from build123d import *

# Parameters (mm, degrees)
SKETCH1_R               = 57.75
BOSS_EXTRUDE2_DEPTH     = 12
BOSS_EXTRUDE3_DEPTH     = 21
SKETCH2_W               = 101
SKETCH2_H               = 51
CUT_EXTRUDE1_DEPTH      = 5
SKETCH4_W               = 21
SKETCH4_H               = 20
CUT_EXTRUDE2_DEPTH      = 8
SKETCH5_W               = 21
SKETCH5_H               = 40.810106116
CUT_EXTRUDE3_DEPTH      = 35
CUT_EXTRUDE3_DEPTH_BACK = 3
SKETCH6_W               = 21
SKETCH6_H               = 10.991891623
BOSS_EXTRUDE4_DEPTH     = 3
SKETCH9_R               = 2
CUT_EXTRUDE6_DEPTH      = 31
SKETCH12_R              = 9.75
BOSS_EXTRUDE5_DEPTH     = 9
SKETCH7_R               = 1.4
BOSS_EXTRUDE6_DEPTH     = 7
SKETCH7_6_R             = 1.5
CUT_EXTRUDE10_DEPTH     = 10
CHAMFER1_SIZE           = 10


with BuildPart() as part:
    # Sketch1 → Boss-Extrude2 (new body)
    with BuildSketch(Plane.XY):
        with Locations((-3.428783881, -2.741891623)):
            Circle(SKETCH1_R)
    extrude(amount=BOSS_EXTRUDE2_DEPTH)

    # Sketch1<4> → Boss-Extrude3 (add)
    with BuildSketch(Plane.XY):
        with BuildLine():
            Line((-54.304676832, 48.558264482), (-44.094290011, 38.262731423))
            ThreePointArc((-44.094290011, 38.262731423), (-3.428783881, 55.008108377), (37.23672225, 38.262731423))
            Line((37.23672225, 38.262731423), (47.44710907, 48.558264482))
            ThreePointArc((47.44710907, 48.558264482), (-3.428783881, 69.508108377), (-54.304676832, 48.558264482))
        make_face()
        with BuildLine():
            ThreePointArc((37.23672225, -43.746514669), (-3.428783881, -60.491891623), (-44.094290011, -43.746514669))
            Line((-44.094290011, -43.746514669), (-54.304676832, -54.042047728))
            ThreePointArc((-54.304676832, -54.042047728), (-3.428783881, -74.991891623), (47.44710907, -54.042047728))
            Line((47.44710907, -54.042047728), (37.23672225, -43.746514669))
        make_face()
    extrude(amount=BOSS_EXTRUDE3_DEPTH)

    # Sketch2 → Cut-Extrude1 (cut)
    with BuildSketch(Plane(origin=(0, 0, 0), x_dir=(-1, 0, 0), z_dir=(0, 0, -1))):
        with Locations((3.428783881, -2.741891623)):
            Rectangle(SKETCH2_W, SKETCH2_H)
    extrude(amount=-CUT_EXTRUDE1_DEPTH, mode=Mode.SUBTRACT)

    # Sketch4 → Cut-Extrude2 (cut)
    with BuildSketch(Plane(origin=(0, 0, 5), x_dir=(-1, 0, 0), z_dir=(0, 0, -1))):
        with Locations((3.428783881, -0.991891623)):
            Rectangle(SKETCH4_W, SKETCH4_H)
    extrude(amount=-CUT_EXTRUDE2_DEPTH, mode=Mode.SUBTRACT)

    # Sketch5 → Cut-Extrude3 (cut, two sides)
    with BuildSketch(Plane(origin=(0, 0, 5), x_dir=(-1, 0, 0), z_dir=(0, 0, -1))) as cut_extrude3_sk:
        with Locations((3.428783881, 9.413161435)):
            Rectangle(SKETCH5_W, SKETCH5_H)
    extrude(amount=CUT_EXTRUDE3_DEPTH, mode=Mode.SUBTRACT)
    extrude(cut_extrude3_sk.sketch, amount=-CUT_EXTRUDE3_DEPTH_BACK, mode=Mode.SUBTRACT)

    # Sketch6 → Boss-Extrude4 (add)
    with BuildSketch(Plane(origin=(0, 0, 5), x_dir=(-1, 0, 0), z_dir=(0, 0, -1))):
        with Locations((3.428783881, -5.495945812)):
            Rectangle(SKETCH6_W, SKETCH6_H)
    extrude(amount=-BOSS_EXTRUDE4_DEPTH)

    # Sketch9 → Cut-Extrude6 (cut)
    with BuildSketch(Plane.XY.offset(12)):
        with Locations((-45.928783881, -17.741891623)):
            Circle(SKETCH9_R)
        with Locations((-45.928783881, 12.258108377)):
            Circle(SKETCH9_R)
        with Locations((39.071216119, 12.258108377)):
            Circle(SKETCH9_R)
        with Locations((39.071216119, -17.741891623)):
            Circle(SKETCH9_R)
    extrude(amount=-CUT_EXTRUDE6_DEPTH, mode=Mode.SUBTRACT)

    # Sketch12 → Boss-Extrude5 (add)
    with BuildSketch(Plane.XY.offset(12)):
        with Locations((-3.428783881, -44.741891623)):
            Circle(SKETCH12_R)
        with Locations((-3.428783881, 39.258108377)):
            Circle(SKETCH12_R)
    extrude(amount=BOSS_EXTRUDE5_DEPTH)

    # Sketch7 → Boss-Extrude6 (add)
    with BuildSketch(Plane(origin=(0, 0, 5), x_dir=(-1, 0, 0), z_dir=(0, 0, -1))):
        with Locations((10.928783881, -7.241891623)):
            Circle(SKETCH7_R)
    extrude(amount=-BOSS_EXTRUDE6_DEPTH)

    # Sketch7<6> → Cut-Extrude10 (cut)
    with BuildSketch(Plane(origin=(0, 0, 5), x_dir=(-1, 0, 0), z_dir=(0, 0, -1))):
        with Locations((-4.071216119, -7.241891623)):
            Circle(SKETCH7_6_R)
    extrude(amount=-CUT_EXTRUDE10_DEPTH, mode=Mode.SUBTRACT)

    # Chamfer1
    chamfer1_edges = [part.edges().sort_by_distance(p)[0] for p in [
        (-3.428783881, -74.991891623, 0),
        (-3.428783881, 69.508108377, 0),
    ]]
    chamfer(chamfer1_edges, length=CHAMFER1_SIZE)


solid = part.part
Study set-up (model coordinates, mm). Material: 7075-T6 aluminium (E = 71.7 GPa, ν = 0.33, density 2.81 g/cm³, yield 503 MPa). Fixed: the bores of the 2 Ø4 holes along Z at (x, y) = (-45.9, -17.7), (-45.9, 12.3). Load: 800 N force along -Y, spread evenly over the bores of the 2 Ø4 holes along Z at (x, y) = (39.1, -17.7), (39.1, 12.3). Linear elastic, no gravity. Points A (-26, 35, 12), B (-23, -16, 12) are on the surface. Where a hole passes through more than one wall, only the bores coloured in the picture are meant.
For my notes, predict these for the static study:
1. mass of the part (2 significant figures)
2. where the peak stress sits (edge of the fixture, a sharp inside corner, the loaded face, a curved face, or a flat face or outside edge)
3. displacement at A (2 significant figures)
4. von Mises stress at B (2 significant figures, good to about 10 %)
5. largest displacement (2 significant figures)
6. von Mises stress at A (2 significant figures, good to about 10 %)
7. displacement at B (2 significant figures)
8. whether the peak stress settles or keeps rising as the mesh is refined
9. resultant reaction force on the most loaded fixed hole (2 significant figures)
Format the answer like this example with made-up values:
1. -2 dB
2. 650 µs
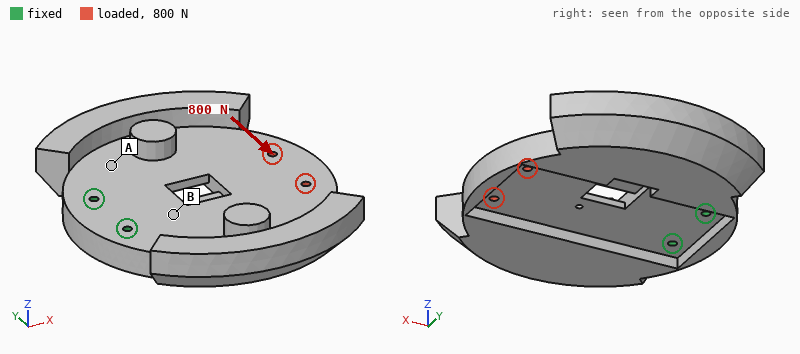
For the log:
1. 430 g
2. edge of the fixture
3. 14 µm
4. 6.3 MPa
5. 39 µm
6. 2.7 MPa
7. 8.4 µm
8. keeps rising
9. 2.1 kN
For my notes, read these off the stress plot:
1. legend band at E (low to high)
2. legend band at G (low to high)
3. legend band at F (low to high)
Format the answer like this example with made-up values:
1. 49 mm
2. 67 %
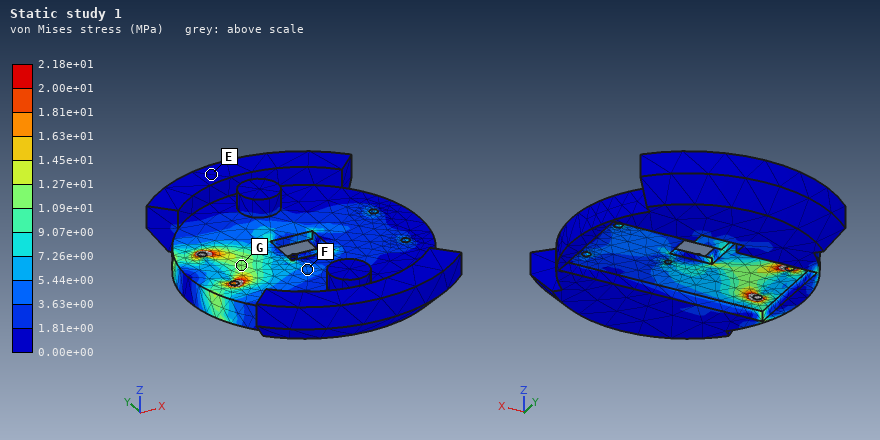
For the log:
1. 0.00e+00 to 1.81e+00 MPa
2. 1.09e+01 to 1.27e+01 MPa
3. 3.63e+00 to 5.44e+00 MPa
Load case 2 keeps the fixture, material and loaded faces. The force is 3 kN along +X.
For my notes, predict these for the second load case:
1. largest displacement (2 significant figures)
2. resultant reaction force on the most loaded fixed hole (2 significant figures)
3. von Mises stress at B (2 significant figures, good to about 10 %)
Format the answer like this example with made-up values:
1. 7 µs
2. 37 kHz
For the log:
1. 18 µm
2. 1.5 kN
3. 9.0 MPa
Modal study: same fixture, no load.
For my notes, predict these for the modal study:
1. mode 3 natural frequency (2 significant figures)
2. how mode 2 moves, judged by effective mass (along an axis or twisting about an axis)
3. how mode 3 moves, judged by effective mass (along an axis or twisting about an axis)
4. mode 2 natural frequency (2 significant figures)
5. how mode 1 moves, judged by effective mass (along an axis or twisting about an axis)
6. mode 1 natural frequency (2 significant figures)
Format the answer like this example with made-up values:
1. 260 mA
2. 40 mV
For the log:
1. 1600 Hz
2. twisting about X
3. along Y
4. 700 Hz
5. along Z
6. 490 Hz
